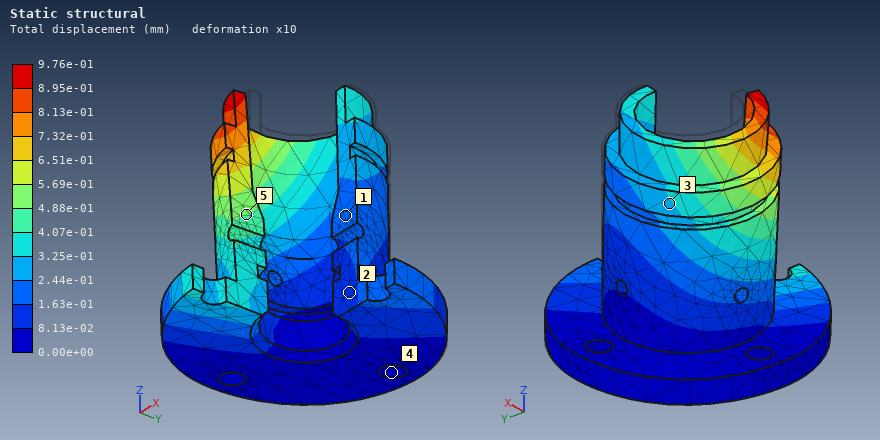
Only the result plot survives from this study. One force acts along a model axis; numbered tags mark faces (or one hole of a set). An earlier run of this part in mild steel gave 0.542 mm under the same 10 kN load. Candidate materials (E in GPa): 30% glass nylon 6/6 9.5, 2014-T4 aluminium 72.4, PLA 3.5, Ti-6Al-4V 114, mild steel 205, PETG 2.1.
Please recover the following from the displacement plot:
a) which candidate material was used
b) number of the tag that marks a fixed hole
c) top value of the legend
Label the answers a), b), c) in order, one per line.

a) Ti-6Al-4V
b) 4
c) 9.76e-01 mm
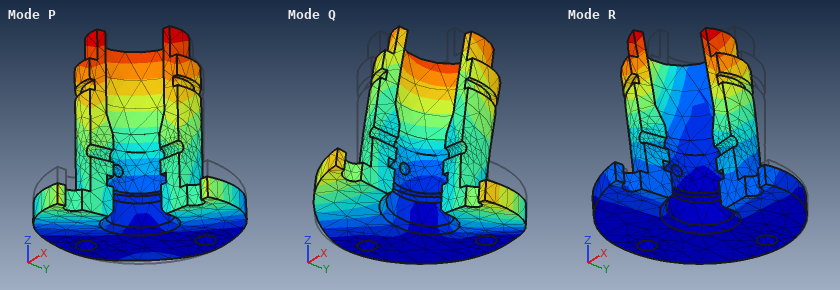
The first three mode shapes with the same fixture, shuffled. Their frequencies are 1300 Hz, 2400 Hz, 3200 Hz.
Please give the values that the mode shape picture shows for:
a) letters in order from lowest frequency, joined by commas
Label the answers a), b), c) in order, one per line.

a) P, R, Q
